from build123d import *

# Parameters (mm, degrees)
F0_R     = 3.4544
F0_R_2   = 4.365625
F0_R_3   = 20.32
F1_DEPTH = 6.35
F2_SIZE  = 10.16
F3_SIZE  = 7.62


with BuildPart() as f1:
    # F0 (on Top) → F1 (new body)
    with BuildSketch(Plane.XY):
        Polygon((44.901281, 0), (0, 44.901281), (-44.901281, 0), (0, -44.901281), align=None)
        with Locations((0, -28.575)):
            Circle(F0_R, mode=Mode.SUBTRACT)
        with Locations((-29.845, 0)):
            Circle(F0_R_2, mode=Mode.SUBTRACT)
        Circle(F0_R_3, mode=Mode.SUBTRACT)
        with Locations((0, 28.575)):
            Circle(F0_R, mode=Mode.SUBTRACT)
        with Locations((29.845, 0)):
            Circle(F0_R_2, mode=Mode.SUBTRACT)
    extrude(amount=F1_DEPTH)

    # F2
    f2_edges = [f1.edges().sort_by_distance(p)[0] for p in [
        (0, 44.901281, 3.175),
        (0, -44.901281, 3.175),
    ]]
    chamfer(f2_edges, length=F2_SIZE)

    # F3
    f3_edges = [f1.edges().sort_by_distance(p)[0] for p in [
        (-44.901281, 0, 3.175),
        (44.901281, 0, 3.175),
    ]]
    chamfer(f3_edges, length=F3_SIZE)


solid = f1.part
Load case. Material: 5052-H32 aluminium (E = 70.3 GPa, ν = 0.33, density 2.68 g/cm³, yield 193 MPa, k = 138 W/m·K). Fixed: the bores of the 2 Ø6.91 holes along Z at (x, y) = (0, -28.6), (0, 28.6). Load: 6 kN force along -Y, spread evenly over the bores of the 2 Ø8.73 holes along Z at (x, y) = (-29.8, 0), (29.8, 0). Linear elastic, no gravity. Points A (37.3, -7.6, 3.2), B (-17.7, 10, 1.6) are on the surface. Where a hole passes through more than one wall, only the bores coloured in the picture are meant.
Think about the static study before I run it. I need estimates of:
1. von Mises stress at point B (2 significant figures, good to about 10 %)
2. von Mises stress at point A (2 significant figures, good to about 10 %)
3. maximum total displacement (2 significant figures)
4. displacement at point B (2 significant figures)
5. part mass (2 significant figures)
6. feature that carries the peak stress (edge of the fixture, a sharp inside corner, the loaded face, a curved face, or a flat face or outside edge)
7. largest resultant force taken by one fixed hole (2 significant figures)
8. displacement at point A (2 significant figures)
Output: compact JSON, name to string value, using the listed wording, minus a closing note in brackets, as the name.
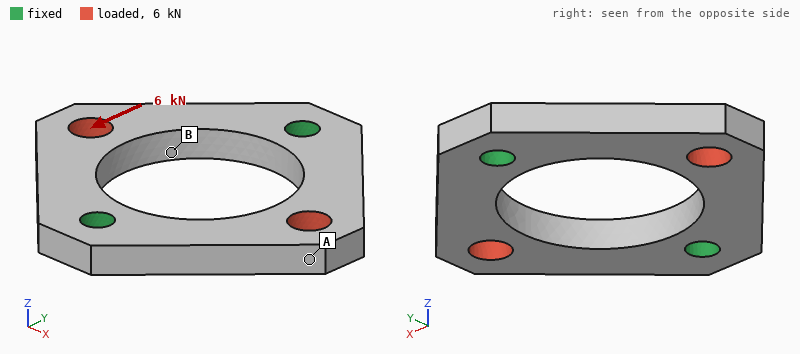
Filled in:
{"von Mises stress at point B": "55 MPa", "von Mises stress at point A": "23 MPa", "maximum total displacement": "29 µm", "displacement at point B": "20 µm", "part mass": "40 g", "feature that carries the peak stress": "the loaded face", "largest resultant force taken by one fixed hole": "3.0 kN", "displacement at point A": "26 µm"}
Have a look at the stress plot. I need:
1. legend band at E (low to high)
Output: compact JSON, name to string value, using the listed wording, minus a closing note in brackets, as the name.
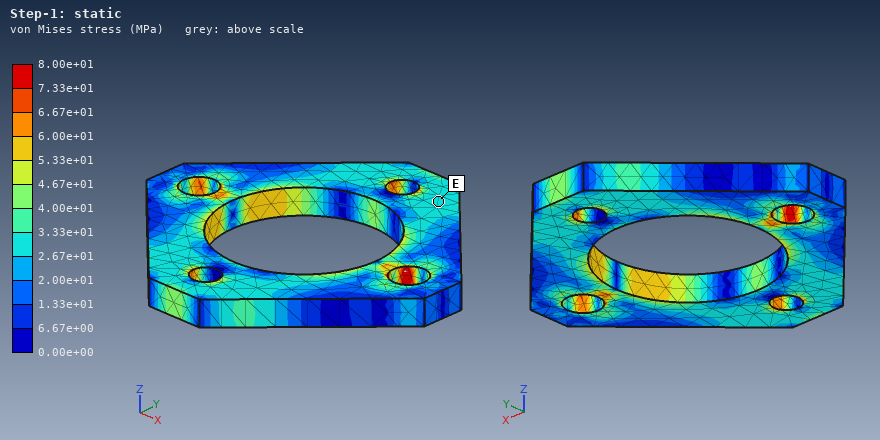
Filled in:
{"legend band at E": "2.67e+01 to 3.33e+01 MPa"}
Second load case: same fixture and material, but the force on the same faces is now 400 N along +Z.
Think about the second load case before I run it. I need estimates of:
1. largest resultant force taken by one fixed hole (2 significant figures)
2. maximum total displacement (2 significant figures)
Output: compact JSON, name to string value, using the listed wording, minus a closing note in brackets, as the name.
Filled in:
{"largest resultant force taken by one fixed hole": "200 N", "maximum total displacement": "78 µm"}
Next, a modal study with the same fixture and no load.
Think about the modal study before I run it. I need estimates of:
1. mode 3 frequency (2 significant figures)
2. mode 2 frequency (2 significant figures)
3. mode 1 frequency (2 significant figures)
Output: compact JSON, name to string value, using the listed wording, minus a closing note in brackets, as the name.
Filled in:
{"mode 3 frequency": "11 kHz", "mode 2 frequency": "3500 Hz", "mode 1 frequency": "3500 Hz"}
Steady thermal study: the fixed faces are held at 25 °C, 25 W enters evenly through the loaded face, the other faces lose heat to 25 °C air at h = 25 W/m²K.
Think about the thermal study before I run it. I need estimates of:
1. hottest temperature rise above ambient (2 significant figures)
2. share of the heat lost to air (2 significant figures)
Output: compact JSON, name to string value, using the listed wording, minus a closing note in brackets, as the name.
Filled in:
{"hottest temperature rise above ambient": "22 K", "share of the heat lost to air": "7.0 %"}
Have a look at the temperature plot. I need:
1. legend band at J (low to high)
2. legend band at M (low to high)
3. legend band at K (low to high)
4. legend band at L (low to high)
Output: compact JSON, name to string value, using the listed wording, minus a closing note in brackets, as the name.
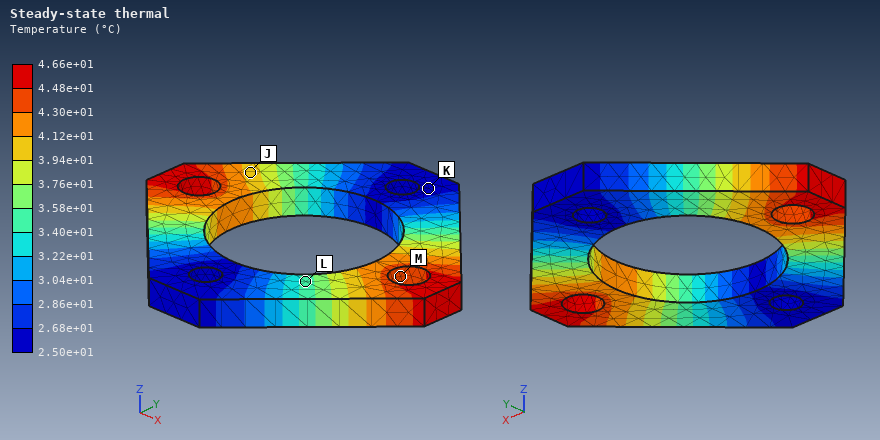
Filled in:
{"legend band at J": "3.94e+01 to 4.12e+01 °C", "legend band at M": "4.30e+01 to 4.48e+01 °C", "legend band at K": "2.50e+01 to 2.68e+01 °C", "legend band at L": "3.40e+01 to 3.58e+01 °C"}
